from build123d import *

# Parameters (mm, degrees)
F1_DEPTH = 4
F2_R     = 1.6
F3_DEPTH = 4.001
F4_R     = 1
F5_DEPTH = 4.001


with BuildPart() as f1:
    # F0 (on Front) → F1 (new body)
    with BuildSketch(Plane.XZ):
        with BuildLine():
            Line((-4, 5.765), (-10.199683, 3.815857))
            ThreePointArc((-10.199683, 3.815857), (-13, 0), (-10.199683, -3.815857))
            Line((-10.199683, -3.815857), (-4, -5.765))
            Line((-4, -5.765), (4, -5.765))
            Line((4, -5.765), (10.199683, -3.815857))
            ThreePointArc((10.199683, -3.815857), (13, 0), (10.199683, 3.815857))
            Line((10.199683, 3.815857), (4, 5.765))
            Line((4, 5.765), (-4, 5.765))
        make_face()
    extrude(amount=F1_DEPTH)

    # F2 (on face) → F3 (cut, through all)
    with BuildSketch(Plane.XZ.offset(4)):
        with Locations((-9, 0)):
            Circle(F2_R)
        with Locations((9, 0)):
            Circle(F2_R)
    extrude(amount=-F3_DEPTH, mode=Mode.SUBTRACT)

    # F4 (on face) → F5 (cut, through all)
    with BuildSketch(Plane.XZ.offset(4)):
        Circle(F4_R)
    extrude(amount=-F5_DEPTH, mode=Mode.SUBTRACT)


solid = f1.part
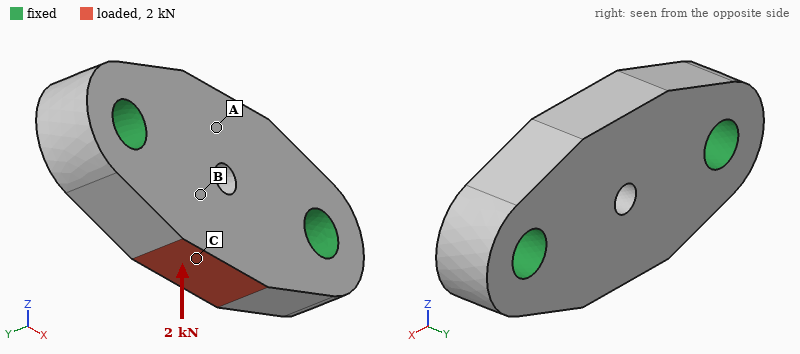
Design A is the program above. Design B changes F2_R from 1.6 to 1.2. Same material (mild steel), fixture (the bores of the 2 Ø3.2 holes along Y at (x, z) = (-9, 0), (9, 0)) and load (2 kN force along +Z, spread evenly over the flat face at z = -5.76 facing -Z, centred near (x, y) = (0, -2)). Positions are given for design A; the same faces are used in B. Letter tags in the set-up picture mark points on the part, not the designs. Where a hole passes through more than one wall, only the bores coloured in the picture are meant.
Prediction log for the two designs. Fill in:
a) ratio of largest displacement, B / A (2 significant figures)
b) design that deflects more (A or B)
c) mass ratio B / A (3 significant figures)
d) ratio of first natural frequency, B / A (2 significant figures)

1.1
B
1.03
0.90
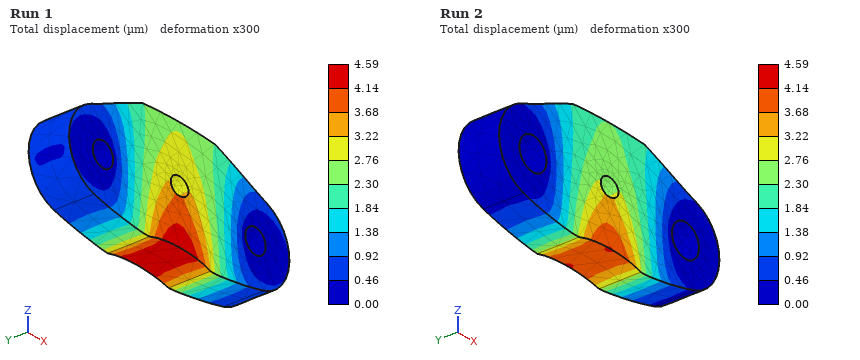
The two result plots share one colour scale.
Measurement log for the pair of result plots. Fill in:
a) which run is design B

Run 1
